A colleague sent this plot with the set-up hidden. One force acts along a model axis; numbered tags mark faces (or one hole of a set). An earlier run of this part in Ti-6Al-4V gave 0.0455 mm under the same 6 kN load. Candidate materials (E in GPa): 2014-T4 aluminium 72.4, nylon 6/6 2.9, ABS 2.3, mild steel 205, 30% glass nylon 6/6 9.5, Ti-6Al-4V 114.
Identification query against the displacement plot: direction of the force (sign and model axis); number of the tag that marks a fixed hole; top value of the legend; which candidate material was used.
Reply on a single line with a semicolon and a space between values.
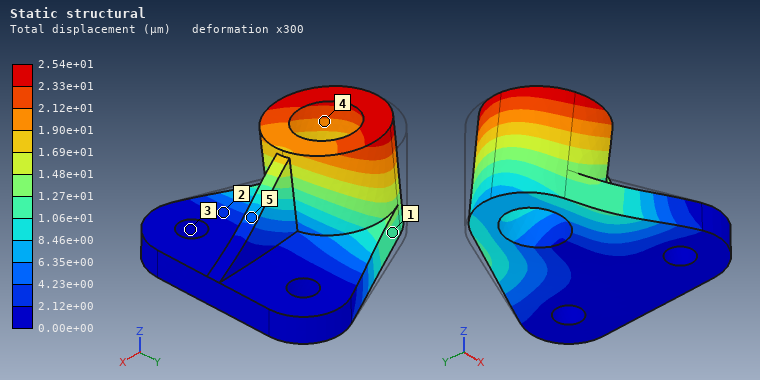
-Y; 3; 2.54e+01 µm; mild steel
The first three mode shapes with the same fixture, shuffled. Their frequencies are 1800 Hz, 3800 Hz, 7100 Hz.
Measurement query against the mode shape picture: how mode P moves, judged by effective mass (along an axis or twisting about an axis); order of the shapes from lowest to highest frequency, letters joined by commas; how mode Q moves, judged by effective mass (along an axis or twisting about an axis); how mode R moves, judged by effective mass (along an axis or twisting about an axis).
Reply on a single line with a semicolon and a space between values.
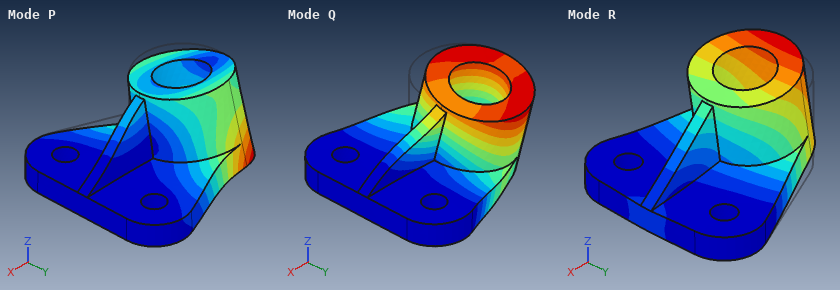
along Y; R, Q, P; along Y; along Z
